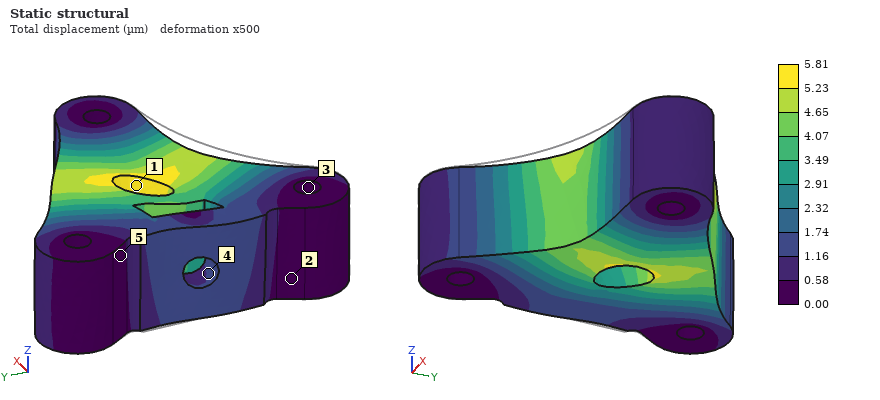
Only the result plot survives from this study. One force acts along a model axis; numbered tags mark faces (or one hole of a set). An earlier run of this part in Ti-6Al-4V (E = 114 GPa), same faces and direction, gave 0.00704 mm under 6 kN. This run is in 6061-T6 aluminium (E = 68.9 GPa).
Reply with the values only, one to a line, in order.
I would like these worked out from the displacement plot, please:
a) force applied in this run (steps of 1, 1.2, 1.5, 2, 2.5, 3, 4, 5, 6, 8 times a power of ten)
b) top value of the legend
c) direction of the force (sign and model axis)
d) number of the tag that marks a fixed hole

3 kN
5.81 µm
+Y
3
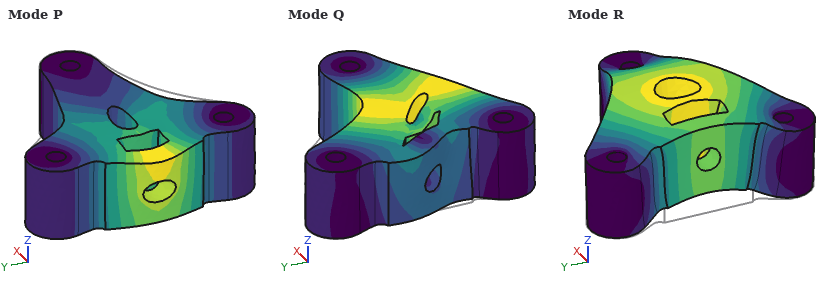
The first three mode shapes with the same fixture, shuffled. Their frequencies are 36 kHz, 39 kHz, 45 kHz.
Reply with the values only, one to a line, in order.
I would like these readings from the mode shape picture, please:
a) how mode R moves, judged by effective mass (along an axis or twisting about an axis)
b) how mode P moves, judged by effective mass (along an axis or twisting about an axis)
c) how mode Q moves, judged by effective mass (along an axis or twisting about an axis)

along Z
along X
along Y
